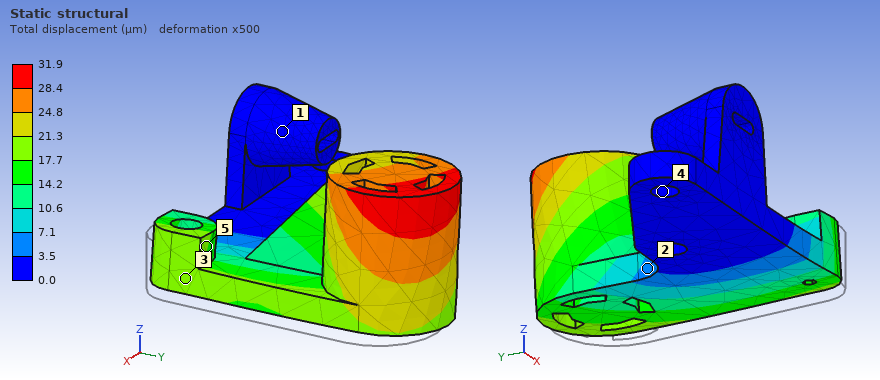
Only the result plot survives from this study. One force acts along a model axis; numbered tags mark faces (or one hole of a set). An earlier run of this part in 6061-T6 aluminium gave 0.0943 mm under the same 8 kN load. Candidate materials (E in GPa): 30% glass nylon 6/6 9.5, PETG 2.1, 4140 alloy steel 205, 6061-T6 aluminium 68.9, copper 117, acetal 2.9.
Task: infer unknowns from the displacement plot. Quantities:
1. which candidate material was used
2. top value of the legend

4140 alloy steel
31.9 µm
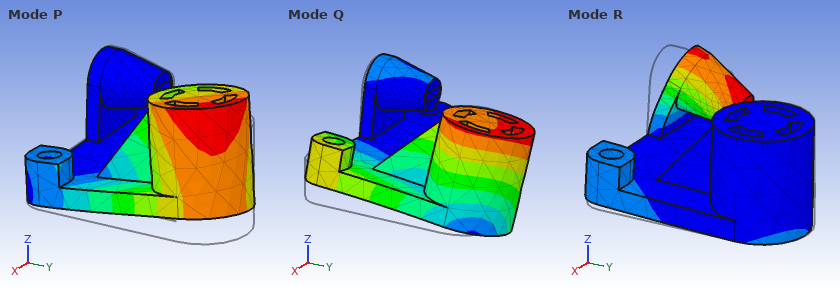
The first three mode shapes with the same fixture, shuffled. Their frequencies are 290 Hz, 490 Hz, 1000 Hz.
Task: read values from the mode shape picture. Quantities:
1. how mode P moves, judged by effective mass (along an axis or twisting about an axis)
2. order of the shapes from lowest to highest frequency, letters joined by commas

along Z
P, Q, R
